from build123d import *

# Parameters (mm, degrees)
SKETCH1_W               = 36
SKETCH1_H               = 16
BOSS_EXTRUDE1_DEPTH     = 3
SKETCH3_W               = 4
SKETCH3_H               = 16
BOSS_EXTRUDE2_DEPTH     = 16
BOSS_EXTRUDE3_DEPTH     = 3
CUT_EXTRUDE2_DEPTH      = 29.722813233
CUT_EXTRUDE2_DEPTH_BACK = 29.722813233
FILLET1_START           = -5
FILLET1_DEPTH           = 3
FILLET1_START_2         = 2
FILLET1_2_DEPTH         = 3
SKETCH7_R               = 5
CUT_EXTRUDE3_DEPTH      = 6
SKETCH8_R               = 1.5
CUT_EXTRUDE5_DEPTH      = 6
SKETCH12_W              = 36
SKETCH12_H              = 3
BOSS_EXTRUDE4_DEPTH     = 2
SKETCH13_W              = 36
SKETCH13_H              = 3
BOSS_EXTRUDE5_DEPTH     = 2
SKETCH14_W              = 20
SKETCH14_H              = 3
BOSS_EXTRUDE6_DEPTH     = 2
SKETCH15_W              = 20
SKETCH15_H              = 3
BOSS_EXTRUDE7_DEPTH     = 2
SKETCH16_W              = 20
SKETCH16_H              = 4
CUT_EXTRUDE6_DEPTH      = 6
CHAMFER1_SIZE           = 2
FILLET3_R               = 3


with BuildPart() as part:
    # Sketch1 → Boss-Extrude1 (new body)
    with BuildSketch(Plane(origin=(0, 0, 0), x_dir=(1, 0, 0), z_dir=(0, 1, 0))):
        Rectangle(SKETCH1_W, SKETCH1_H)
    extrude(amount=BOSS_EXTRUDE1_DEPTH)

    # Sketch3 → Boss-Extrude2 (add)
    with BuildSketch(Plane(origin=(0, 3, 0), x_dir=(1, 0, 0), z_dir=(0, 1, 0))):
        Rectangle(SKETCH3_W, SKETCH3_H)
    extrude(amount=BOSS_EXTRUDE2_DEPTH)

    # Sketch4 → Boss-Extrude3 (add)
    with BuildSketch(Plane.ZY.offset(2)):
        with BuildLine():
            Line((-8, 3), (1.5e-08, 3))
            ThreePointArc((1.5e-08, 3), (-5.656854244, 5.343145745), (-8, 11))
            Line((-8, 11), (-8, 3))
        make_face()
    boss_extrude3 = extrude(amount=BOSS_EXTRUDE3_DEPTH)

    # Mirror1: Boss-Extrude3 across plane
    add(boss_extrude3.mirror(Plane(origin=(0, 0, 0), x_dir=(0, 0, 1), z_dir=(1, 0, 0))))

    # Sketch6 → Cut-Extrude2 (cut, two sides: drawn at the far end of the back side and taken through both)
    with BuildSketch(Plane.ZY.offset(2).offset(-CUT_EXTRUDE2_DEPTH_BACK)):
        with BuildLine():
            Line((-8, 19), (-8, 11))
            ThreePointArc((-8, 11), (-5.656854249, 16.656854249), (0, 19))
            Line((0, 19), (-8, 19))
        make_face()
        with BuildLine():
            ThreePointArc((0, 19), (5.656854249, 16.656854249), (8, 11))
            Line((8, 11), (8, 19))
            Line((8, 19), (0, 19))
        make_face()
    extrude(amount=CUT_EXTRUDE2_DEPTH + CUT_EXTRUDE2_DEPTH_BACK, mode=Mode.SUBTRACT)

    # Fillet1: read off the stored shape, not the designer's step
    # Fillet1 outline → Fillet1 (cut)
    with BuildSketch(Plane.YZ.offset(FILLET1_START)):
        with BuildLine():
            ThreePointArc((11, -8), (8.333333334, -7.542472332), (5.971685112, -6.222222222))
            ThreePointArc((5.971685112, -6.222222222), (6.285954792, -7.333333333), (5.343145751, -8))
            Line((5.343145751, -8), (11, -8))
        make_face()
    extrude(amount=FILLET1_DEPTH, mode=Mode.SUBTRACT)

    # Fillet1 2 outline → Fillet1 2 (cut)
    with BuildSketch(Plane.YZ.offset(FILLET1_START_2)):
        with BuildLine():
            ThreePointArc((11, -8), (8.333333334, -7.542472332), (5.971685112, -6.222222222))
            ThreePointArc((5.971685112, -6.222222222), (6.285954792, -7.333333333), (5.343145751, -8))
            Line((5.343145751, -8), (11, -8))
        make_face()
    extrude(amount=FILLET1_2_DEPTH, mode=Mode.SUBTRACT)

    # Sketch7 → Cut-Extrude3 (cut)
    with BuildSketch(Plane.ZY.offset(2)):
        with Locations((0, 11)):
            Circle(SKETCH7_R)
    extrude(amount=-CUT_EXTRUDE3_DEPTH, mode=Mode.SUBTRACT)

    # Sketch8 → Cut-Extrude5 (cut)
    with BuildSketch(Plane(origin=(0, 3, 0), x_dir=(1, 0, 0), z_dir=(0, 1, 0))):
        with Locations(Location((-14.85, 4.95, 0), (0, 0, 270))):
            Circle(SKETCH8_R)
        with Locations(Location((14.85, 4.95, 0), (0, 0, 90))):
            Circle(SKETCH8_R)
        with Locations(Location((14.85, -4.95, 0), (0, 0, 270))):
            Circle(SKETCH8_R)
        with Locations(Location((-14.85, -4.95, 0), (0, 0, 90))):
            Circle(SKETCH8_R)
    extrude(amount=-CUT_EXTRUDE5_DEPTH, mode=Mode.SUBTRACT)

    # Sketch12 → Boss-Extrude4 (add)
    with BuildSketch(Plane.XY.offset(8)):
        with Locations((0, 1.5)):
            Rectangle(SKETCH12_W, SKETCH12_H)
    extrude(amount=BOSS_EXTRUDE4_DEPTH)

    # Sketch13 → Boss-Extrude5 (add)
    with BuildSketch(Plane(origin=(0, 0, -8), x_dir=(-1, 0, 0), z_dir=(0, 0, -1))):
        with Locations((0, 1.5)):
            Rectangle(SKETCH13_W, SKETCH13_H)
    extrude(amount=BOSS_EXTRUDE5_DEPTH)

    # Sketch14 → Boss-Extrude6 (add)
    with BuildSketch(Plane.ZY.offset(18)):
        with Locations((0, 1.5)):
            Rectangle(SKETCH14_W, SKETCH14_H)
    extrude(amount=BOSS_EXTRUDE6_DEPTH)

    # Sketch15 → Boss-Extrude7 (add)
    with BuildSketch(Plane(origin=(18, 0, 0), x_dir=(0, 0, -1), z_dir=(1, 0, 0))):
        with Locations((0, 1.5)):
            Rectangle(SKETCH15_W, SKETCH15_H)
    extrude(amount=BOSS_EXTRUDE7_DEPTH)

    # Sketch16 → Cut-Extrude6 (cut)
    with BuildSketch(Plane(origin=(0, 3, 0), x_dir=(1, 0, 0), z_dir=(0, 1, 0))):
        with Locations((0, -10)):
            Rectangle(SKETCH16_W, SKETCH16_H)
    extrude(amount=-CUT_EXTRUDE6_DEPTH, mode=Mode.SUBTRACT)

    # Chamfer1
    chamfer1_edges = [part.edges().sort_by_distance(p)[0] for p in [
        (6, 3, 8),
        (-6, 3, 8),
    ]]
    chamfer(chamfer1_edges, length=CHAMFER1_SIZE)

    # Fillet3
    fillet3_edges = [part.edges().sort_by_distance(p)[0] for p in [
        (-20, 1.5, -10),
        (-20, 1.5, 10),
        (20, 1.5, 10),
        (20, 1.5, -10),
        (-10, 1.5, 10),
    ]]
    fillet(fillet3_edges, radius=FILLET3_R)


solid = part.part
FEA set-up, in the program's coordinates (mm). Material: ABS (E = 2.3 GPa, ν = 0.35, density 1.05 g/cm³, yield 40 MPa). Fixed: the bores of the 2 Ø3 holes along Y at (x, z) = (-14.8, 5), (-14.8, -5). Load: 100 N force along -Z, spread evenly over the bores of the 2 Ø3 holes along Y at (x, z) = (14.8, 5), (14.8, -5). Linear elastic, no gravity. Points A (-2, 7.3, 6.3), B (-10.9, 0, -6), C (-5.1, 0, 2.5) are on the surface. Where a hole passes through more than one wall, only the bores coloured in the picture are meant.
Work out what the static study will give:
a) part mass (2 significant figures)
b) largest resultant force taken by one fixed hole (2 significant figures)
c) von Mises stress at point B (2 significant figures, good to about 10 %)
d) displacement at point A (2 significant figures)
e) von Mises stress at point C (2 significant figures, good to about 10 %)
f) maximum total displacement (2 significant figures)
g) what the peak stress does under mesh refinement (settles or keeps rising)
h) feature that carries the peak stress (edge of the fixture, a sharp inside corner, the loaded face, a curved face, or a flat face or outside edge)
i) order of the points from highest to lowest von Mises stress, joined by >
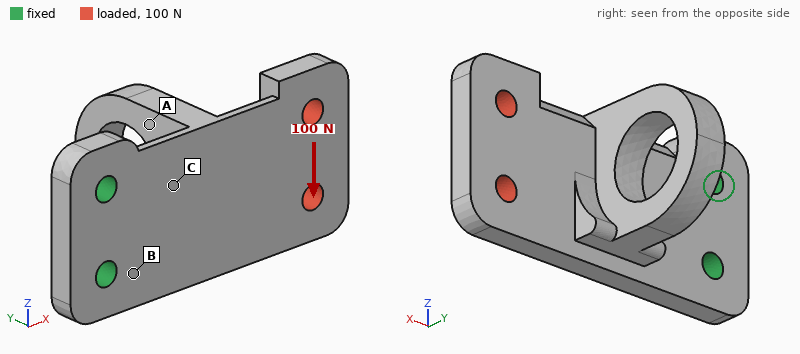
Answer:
2.9 g
260 N
12 MPa
0.15 mm
7.3 MPa
0.49 mm
keeps rising
edge of the fixture
B > C > A
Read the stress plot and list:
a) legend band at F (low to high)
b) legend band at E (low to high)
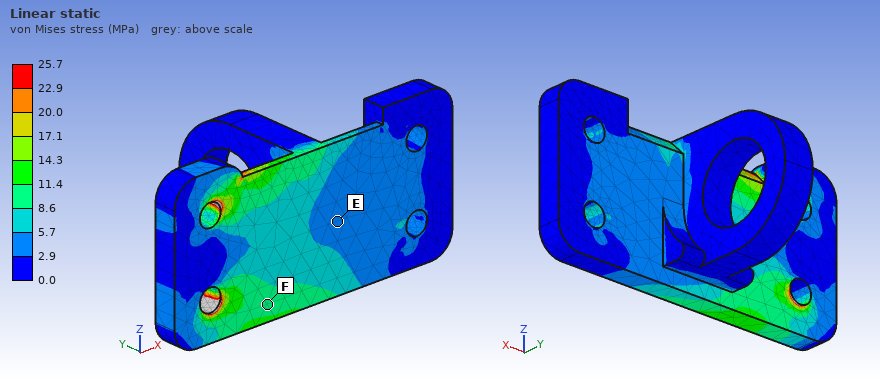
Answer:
8.6 to 11.4 MPa
2.9 to 5.7 MPa
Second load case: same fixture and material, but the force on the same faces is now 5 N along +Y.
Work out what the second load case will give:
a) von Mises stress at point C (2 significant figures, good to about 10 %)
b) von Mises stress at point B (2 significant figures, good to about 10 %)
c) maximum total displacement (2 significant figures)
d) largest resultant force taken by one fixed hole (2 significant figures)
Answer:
3.2 MPa
4.7 MPa
0.50 mm
2.7 N
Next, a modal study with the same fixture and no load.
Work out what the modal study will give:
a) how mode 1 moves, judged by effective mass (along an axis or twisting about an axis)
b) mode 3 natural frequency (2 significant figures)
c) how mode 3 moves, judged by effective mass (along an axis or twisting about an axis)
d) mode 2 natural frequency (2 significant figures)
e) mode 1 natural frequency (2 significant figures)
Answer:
along Y
2700 Hz
along Z
1800 Hz
580 Hz
